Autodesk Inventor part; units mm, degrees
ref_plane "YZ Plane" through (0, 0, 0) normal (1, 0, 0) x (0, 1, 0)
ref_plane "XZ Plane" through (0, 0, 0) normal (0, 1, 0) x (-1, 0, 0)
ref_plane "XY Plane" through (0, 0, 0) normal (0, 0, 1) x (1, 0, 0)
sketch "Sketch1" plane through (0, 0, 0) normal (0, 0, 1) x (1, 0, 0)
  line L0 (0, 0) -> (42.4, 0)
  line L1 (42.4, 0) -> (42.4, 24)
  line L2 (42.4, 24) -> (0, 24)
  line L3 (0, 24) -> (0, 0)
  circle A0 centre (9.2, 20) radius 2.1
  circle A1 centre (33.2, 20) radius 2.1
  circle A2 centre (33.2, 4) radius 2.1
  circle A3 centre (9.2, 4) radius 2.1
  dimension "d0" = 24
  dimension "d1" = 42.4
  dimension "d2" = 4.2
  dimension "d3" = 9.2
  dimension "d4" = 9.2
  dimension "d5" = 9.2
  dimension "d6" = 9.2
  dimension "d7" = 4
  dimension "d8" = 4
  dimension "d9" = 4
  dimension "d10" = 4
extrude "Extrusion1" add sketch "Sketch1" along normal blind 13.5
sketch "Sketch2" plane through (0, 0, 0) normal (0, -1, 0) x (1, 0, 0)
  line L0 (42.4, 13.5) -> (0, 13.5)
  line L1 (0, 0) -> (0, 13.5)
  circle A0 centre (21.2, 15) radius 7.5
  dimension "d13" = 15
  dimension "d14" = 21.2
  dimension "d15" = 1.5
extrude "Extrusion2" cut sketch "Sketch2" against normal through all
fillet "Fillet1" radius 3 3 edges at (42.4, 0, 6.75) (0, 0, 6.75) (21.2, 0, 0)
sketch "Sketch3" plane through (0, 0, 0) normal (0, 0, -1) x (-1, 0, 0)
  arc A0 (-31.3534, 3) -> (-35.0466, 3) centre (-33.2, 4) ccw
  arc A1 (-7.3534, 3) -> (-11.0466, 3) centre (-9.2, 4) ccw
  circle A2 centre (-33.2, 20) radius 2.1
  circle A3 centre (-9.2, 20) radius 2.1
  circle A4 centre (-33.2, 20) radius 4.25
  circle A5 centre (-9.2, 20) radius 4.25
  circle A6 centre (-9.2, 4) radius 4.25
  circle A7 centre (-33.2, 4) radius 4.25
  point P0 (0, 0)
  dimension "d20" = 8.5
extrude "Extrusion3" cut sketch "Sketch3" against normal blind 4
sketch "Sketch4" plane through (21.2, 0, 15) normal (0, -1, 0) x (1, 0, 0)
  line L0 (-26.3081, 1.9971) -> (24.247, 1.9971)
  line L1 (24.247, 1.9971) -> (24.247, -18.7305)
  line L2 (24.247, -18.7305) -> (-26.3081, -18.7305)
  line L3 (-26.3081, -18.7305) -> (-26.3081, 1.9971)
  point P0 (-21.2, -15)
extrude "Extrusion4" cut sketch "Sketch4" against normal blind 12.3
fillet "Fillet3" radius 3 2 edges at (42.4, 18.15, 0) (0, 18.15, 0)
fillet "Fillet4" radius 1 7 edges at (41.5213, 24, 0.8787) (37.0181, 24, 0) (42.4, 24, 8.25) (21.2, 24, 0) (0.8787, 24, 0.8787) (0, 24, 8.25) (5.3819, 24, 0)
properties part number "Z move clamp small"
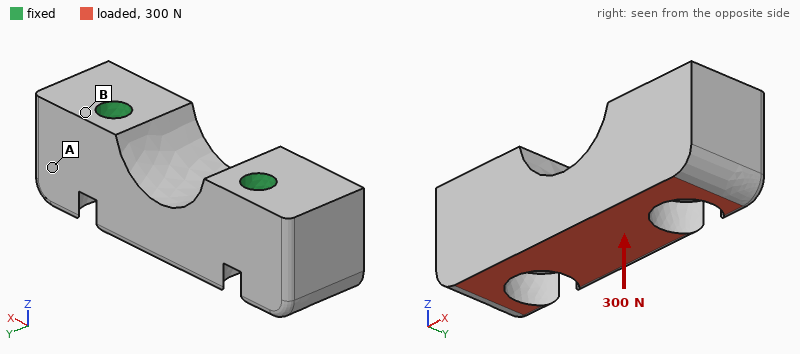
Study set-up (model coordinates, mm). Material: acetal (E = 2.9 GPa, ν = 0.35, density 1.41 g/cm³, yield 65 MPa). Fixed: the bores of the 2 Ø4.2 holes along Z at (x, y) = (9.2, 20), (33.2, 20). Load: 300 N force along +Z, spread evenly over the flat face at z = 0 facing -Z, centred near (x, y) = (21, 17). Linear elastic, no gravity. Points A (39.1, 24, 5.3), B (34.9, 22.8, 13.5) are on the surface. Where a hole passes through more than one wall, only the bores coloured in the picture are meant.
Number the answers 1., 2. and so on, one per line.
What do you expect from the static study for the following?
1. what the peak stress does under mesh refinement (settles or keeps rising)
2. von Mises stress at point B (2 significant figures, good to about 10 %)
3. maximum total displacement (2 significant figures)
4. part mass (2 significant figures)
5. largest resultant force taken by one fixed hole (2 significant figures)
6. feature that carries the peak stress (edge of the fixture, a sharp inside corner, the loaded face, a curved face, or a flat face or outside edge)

1. keeps rising
2. 0.91 MPa
3. 18 µm
4. 7.3 g
5. 160 N
6. edge of the fixture
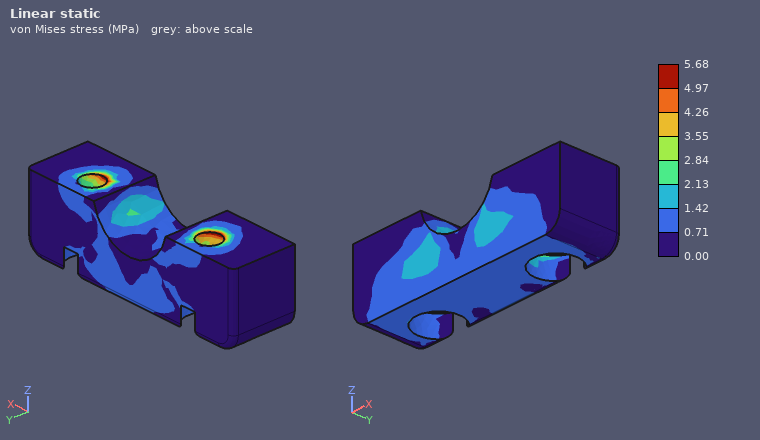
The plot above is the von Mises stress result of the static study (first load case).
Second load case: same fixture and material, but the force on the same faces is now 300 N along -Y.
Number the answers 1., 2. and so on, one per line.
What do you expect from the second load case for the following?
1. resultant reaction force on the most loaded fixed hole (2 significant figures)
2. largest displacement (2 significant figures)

1. 150 N
2. 51 µm
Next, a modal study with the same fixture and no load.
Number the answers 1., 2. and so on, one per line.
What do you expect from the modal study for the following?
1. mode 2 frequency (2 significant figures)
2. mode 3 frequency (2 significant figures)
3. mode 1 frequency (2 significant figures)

1. 12 kHz
2. 12 kHz
3. 10 kHz
